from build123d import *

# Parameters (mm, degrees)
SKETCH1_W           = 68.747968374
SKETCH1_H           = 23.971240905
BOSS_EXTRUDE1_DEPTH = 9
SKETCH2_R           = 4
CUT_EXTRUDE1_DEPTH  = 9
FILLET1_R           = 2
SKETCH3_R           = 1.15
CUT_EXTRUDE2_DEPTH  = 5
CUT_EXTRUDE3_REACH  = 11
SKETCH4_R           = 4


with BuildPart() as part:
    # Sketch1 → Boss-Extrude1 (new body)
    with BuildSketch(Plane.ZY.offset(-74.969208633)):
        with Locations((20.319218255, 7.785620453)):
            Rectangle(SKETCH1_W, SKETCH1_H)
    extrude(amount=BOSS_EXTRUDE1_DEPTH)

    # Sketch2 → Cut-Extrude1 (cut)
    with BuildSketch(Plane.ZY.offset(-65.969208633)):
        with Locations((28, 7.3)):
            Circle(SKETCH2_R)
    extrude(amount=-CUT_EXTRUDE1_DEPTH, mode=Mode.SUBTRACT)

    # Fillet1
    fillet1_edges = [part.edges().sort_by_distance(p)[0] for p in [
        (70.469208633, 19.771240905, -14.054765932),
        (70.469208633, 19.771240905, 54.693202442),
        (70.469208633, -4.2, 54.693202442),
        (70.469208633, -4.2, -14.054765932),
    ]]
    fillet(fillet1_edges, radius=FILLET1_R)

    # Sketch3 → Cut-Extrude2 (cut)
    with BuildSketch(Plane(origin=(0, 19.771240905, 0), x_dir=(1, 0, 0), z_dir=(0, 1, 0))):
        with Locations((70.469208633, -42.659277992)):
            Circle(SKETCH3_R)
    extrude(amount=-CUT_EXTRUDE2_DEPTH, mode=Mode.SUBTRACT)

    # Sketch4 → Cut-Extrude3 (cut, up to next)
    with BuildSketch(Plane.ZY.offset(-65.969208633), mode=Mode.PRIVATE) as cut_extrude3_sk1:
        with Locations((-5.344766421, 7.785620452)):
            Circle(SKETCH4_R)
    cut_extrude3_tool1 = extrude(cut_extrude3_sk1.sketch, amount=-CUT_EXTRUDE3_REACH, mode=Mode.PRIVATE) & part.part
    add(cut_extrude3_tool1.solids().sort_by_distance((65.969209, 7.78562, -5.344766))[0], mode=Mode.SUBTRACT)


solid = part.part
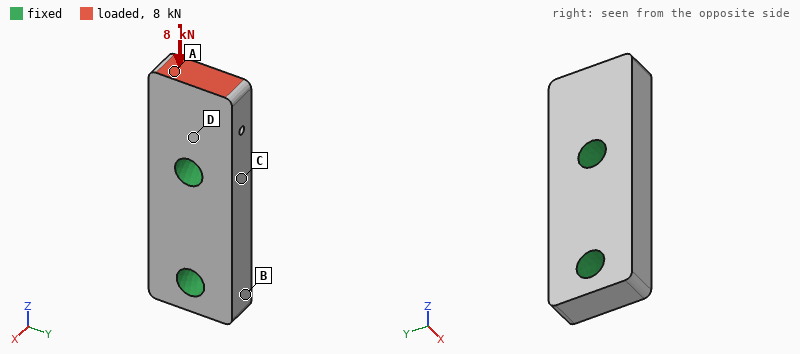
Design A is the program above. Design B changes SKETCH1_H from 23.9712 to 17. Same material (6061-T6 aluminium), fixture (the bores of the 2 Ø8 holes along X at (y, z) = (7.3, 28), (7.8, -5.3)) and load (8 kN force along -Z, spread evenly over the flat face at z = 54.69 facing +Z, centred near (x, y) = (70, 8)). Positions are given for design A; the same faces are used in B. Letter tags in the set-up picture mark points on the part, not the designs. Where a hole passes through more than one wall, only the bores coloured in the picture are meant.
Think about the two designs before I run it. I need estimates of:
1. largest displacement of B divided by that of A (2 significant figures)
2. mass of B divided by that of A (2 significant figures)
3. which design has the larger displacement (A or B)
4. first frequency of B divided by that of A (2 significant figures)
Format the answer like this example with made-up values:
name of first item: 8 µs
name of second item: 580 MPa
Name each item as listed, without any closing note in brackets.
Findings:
largest displacement of B divided by that of A: 1.3
mass of B divided by that of A: 0.69
which design has the larger displacement: B
first frequency of B divided by that of A: 1.1
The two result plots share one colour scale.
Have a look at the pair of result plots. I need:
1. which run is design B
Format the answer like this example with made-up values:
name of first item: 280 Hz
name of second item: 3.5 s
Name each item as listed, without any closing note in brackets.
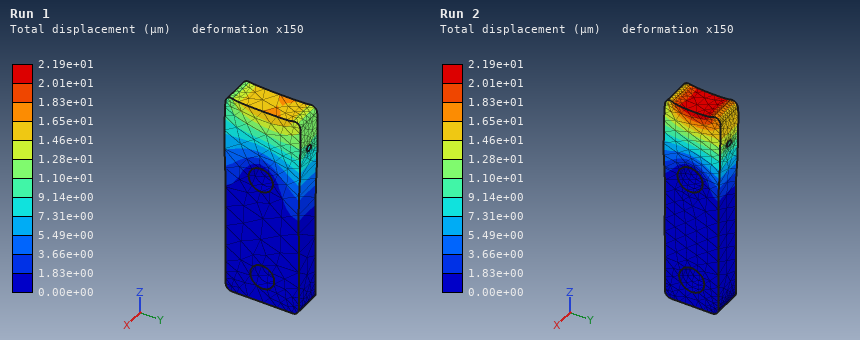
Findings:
which run is design B: Run 2
